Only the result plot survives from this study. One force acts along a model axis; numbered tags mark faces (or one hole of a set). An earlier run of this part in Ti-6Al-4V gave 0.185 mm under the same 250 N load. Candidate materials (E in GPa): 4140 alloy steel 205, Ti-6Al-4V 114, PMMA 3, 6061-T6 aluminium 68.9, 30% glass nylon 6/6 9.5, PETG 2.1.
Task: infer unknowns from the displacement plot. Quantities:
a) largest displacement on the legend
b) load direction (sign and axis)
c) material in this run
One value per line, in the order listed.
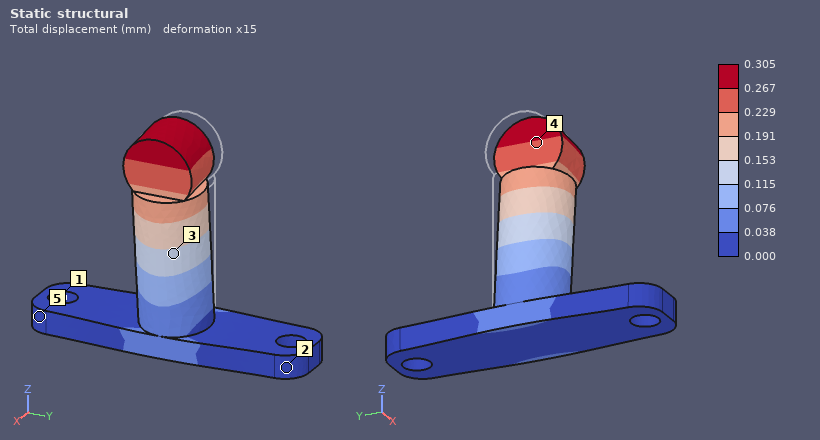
0.305 mm
+X
6061-T6 aluminium
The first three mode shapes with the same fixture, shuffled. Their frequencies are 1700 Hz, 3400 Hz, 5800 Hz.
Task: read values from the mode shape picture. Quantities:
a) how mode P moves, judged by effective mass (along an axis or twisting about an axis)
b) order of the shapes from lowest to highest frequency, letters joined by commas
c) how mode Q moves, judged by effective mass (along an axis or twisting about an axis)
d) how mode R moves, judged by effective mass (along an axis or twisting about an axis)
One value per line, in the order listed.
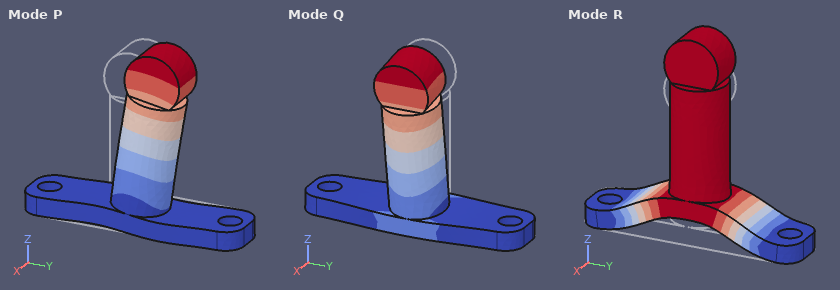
along Y
Q, P, R
along X
along Z
